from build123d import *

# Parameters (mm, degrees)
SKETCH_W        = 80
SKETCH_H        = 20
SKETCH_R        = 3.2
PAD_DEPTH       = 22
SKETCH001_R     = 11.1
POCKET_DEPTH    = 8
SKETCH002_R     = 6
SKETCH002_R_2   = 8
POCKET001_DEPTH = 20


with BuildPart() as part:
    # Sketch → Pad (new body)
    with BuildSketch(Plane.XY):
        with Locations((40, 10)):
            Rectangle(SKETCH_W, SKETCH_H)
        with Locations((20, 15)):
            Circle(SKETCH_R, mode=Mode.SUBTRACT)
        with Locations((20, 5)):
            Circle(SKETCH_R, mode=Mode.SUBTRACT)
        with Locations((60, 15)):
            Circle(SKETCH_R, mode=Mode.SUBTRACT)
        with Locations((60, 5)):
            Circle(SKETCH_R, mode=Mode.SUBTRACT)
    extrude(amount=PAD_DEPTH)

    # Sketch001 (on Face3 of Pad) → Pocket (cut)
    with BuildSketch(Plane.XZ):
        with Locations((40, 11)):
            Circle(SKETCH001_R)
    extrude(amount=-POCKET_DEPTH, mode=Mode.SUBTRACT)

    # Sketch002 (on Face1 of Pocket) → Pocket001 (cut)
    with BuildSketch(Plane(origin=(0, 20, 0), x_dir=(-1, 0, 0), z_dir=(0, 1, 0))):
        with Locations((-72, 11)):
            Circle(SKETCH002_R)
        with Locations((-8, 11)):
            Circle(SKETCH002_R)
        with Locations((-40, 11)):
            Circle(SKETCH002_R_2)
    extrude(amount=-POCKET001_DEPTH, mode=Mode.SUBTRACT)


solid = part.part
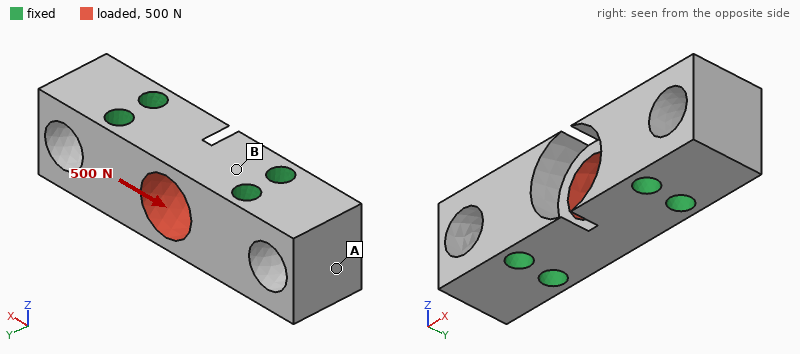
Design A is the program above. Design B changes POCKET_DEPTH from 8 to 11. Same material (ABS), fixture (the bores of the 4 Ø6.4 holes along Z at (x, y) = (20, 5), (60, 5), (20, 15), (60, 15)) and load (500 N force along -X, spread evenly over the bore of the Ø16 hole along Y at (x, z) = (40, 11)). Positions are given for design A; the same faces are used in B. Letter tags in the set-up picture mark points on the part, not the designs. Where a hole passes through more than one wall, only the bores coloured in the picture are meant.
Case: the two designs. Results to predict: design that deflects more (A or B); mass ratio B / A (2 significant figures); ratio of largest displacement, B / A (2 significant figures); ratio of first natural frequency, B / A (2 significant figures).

B
0.98
1.3
1.00
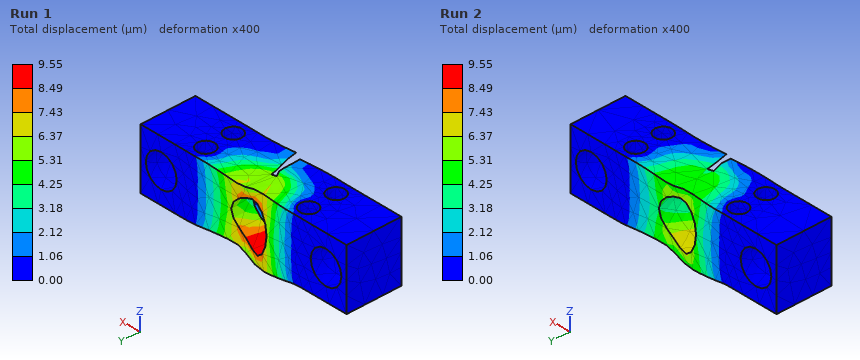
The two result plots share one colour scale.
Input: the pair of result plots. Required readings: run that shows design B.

Run 1
